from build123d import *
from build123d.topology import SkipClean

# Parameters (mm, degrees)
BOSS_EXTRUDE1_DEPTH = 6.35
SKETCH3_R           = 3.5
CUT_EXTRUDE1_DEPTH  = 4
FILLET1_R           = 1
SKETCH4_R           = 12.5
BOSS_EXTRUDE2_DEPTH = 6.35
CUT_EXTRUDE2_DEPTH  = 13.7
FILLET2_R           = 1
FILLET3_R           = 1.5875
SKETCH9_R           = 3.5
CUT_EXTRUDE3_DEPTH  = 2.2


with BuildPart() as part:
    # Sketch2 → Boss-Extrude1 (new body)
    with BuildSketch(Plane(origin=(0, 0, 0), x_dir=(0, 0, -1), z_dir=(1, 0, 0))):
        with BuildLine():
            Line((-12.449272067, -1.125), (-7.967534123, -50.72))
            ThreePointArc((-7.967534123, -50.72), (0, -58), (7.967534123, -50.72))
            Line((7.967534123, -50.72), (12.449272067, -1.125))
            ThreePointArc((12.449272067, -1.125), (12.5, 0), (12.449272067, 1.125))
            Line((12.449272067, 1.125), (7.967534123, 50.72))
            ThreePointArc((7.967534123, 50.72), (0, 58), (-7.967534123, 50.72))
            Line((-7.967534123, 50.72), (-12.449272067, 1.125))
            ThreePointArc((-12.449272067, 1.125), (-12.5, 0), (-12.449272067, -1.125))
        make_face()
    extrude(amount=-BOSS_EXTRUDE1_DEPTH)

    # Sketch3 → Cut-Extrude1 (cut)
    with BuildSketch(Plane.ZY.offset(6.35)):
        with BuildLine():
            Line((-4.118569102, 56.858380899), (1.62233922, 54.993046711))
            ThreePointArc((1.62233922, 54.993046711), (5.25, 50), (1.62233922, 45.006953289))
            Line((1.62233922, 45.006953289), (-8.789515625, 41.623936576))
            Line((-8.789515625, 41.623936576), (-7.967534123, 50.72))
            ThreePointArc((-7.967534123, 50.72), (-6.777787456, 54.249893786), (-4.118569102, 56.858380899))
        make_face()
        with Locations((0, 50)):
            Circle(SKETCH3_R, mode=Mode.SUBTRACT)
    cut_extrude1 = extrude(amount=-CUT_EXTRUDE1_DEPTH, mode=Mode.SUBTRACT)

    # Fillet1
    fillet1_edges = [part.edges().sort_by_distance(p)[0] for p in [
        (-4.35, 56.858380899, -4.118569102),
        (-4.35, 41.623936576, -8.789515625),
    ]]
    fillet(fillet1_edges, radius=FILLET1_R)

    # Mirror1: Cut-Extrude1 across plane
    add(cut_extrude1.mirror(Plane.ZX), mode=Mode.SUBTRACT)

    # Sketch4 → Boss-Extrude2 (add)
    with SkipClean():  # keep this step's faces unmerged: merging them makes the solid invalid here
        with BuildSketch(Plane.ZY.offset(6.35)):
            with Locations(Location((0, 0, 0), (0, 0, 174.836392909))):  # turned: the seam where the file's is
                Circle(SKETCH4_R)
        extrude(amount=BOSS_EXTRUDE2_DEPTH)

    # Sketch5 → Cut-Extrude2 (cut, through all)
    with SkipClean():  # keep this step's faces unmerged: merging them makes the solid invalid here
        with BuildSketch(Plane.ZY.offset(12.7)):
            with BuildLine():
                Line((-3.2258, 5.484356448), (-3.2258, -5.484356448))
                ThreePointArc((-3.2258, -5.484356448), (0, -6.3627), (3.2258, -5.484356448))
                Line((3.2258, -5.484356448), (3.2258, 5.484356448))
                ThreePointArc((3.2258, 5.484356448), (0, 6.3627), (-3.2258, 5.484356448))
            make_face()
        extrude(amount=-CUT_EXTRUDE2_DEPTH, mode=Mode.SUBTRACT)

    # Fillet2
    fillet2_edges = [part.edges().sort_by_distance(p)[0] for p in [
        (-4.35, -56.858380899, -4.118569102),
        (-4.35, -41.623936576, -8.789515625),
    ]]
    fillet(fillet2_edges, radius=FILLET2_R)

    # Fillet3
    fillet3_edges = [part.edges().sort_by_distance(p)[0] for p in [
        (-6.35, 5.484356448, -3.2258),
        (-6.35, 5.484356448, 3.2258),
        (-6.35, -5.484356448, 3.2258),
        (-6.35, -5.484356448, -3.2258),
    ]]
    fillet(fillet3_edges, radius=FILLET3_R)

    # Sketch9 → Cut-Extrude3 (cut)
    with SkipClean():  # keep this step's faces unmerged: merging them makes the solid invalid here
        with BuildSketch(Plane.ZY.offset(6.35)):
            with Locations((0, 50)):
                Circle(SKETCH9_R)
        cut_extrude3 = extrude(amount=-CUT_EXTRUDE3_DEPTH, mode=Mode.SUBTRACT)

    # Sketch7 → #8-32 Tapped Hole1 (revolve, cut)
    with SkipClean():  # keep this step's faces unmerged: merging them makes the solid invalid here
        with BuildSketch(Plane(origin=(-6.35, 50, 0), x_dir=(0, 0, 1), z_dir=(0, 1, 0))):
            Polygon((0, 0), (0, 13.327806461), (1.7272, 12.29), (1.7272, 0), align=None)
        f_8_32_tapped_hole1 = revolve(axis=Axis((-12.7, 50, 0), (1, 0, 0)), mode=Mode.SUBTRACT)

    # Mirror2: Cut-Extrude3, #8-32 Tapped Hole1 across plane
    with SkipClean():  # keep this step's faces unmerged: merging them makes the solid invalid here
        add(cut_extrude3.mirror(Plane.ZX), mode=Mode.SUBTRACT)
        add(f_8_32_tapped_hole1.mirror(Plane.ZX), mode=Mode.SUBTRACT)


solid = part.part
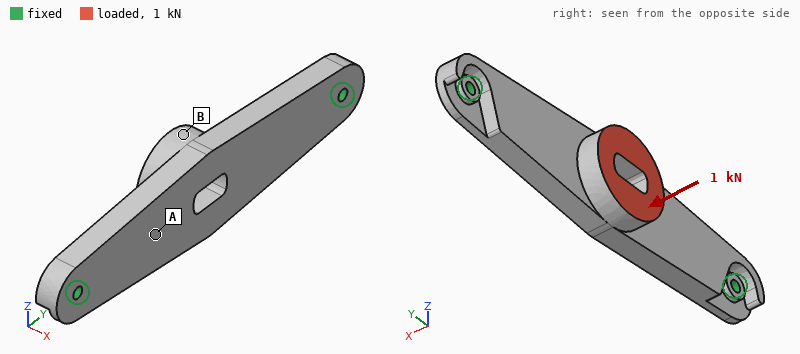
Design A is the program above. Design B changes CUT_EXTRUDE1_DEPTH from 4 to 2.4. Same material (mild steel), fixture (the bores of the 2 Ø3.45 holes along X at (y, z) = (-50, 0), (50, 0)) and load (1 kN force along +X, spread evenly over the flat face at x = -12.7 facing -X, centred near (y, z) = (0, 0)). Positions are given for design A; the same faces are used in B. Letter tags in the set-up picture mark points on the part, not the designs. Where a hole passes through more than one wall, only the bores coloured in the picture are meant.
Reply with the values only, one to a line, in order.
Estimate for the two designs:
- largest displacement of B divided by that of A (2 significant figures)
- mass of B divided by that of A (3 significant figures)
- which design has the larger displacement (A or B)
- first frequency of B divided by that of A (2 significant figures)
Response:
0.89
1.02
A
1.1
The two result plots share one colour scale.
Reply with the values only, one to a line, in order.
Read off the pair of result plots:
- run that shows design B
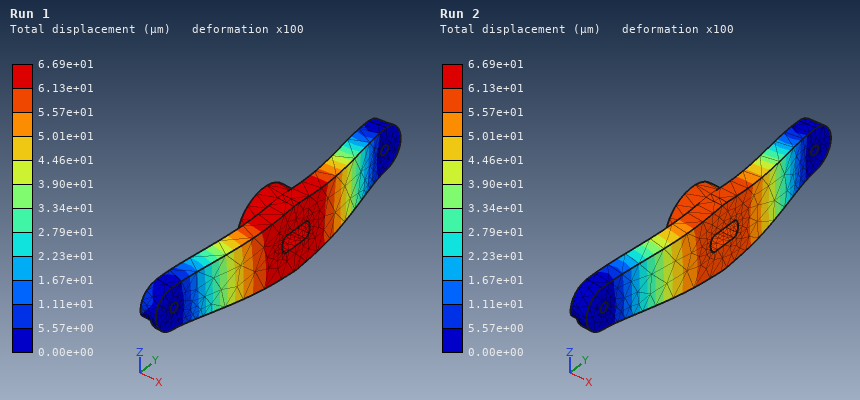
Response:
Run 2
